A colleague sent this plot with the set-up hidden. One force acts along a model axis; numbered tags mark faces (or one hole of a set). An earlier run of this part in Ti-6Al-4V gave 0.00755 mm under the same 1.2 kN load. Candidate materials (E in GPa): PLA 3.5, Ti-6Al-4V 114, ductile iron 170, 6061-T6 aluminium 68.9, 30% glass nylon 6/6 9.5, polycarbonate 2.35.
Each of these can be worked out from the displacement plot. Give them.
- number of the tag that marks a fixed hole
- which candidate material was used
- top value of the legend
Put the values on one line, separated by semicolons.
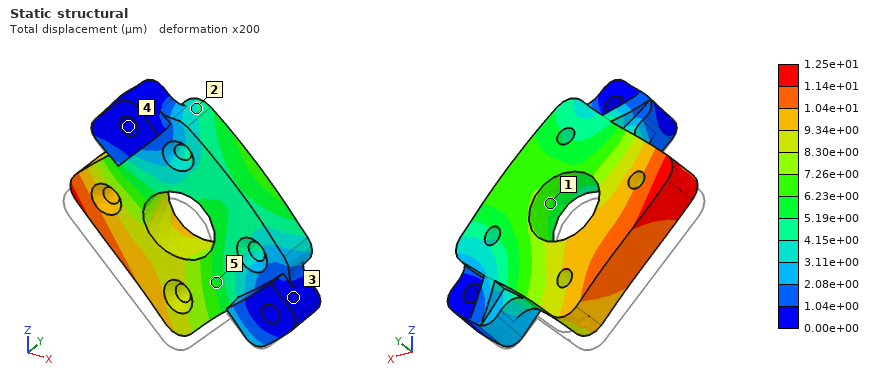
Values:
4; 6061-T6 aluminium; 1.25e+01 µm
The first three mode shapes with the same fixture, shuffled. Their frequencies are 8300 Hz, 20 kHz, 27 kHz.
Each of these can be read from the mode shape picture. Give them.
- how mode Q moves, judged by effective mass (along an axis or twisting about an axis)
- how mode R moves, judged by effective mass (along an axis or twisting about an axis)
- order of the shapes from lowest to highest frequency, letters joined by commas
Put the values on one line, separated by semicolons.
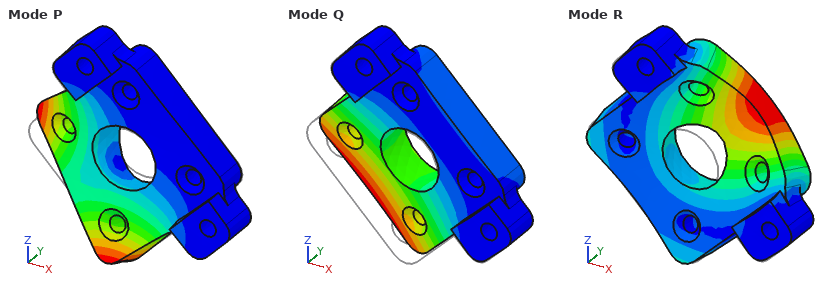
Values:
along Y; along Y; Q, P, R
